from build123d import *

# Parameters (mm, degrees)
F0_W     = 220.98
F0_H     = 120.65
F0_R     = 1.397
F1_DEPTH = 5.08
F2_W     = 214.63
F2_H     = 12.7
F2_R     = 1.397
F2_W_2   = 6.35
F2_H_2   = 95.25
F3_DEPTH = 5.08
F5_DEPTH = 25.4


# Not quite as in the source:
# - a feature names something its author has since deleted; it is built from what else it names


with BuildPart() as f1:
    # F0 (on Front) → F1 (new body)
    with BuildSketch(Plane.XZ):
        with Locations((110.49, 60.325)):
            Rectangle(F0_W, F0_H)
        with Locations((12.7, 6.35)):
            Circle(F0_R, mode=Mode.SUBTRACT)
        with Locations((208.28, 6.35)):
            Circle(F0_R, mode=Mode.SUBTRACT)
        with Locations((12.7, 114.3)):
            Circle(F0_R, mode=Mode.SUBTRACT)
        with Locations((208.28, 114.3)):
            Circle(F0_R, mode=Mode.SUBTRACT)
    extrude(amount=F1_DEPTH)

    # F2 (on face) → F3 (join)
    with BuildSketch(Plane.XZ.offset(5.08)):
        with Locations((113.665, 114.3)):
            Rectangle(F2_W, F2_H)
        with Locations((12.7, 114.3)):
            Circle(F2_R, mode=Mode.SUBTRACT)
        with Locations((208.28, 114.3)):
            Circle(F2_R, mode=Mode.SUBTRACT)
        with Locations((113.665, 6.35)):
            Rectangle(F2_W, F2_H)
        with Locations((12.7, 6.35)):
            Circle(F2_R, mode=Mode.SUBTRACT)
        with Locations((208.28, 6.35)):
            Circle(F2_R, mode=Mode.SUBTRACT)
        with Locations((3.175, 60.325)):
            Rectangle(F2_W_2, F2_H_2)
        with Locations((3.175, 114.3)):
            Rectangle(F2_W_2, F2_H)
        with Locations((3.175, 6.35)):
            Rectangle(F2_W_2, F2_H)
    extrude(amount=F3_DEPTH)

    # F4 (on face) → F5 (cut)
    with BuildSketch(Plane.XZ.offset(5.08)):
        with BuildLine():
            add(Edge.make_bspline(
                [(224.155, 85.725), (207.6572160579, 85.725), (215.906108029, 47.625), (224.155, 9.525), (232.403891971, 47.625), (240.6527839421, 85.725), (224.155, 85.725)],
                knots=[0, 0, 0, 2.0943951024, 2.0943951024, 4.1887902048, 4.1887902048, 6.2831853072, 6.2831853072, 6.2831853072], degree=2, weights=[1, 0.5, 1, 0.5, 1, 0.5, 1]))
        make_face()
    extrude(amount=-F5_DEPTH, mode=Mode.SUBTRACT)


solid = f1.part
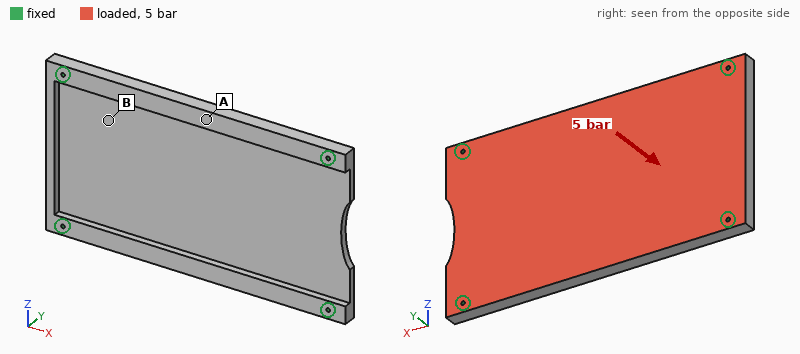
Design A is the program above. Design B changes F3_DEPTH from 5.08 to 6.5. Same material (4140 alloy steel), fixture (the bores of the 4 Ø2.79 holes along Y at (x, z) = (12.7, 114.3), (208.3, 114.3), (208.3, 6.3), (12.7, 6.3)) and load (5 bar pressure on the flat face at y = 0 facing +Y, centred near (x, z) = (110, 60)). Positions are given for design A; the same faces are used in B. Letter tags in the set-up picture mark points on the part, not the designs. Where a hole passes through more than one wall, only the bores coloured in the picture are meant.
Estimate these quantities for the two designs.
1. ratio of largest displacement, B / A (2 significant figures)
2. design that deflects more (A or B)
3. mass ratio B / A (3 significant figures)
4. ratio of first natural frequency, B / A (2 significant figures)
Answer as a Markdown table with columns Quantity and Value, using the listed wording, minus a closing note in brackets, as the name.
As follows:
| Quantity | Value |
|---|---|
| ratio of largest displacement, B / A | 0.79 |
| design that deflects more | A |
| mass ratio B / A | 1.05 |
| ratio of first natural frequency, B / A | 1.1 |
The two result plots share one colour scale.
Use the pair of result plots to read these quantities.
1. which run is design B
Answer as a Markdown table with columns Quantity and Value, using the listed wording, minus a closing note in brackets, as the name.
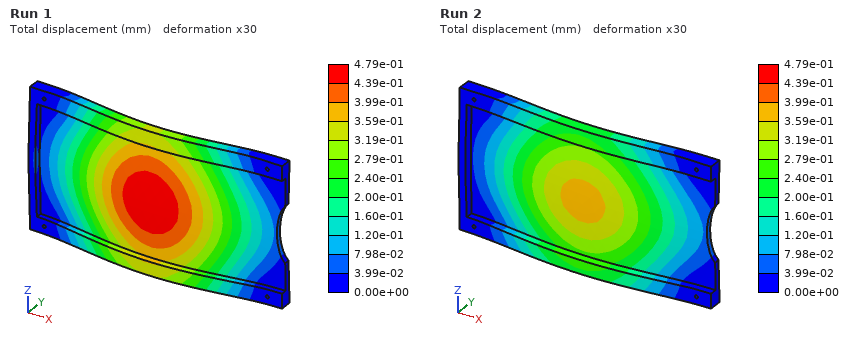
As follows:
| Quantity | Value |
|---|---|
| which run is design B | Run 2 |
